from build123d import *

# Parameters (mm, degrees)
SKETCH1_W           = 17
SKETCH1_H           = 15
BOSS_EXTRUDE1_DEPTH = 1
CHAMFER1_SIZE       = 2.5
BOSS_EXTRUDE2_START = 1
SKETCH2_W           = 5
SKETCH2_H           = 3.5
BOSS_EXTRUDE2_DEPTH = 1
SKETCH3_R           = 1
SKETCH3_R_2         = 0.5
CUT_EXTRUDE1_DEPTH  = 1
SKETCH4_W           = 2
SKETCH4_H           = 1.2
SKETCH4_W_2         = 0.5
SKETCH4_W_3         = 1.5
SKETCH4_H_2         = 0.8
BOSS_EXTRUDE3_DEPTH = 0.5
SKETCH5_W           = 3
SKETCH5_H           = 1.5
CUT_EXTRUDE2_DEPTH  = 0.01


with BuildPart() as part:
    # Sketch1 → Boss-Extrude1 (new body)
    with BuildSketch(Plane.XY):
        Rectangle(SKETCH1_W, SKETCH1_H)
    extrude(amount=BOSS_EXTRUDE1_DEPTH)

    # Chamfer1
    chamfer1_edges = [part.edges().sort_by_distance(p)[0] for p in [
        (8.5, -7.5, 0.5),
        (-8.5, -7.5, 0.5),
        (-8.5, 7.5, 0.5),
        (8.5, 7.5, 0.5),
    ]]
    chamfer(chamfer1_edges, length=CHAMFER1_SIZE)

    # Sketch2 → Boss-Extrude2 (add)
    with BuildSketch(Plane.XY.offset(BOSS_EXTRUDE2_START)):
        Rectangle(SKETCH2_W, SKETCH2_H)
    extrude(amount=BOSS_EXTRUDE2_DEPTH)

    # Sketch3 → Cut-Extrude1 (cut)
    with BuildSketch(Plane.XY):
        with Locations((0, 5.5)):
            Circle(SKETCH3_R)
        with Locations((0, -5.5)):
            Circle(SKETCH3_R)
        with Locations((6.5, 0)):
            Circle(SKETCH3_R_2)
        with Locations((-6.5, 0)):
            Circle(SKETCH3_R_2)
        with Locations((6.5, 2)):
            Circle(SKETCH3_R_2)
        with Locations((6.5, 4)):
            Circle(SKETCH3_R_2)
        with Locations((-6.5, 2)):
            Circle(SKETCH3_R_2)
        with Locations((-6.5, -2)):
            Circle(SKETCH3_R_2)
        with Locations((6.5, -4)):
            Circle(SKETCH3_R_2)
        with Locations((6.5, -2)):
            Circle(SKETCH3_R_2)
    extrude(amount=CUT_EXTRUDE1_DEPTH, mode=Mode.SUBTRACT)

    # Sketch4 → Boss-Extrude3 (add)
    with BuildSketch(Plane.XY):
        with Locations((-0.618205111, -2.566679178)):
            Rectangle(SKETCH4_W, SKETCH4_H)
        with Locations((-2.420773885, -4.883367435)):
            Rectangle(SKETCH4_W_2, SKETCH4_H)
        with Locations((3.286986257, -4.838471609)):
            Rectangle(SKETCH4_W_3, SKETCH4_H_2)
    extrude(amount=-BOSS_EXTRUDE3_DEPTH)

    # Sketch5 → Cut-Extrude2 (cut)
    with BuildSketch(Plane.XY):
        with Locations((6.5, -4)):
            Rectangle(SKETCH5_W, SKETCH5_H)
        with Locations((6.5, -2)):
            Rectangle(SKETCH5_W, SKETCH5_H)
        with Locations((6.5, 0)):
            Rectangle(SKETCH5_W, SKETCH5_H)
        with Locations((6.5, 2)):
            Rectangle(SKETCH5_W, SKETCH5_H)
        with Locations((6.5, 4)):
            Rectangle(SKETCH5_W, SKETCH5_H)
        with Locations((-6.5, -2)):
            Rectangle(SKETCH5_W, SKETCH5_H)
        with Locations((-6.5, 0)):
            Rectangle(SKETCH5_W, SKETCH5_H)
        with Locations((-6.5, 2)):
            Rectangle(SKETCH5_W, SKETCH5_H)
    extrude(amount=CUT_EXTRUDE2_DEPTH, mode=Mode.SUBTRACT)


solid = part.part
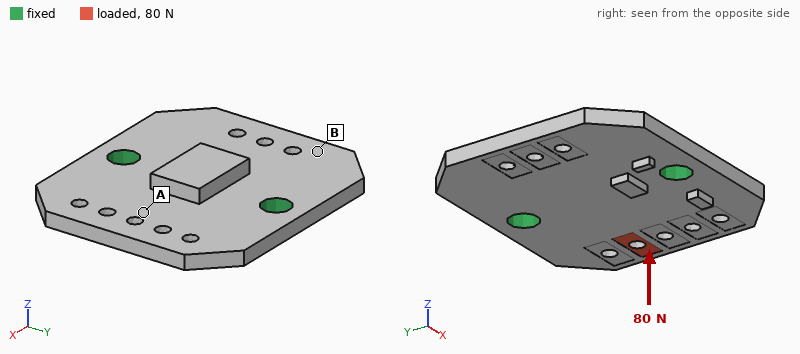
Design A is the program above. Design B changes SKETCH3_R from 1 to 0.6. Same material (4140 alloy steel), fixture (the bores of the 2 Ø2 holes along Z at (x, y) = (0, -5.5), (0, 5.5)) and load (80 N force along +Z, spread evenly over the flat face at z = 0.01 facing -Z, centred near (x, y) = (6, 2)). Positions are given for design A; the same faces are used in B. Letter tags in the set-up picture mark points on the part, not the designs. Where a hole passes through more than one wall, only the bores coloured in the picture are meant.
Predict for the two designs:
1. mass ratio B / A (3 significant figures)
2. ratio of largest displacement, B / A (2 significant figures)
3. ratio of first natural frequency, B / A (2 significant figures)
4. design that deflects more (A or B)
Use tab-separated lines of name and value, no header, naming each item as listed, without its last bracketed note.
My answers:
mass ratio B / A	1.02
ratio of largest displacement, B / A	1.2
ratio of first natural frequency, B / A	0.83
design that deflects more	B
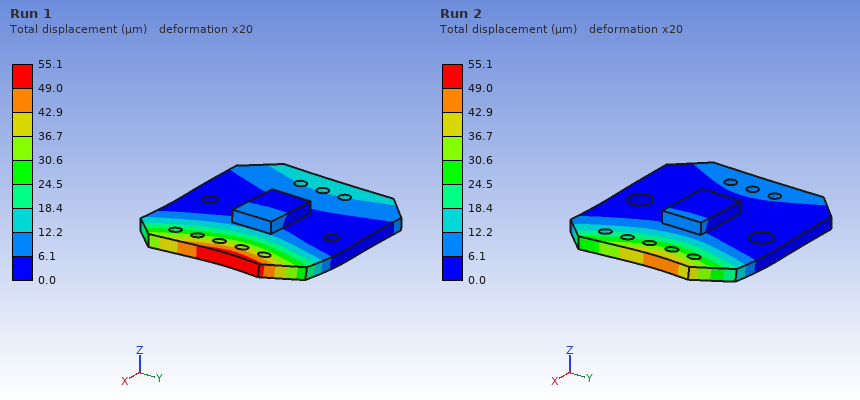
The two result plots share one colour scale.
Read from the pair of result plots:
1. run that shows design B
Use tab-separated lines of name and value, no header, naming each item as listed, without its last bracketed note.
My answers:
run that shows design B	Run 1
